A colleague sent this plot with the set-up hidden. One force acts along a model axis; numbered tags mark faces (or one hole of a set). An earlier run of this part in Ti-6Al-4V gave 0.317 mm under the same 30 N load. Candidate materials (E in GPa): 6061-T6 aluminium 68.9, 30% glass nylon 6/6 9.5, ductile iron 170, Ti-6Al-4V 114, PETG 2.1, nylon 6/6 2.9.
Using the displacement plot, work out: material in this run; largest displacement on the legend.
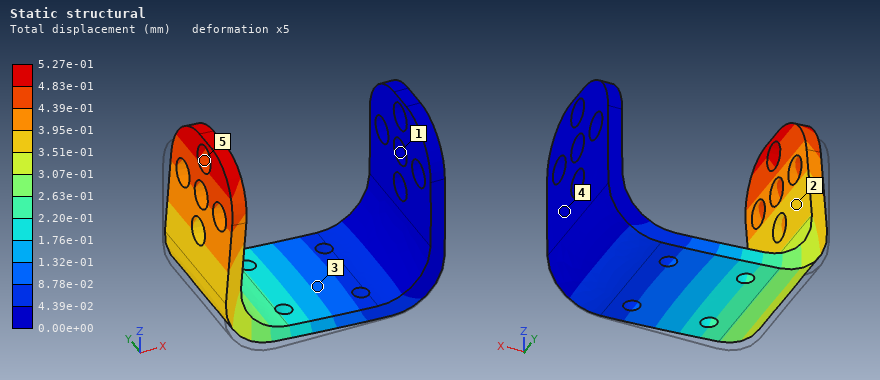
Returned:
6061-T6 aluminium
5.27e-01 mm
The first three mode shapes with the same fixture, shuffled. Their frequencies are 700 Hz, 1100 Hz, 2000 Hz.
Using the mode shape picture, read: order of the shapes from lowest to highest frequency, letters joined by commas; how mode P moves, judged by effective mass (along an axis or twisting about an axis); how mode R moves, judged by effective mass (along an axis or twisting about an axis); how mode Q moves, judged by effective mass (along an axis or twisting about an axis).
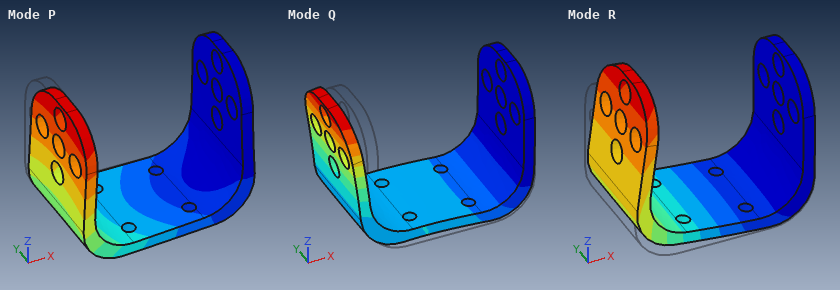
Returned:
R, P, Q
along Y
along Z
along X
